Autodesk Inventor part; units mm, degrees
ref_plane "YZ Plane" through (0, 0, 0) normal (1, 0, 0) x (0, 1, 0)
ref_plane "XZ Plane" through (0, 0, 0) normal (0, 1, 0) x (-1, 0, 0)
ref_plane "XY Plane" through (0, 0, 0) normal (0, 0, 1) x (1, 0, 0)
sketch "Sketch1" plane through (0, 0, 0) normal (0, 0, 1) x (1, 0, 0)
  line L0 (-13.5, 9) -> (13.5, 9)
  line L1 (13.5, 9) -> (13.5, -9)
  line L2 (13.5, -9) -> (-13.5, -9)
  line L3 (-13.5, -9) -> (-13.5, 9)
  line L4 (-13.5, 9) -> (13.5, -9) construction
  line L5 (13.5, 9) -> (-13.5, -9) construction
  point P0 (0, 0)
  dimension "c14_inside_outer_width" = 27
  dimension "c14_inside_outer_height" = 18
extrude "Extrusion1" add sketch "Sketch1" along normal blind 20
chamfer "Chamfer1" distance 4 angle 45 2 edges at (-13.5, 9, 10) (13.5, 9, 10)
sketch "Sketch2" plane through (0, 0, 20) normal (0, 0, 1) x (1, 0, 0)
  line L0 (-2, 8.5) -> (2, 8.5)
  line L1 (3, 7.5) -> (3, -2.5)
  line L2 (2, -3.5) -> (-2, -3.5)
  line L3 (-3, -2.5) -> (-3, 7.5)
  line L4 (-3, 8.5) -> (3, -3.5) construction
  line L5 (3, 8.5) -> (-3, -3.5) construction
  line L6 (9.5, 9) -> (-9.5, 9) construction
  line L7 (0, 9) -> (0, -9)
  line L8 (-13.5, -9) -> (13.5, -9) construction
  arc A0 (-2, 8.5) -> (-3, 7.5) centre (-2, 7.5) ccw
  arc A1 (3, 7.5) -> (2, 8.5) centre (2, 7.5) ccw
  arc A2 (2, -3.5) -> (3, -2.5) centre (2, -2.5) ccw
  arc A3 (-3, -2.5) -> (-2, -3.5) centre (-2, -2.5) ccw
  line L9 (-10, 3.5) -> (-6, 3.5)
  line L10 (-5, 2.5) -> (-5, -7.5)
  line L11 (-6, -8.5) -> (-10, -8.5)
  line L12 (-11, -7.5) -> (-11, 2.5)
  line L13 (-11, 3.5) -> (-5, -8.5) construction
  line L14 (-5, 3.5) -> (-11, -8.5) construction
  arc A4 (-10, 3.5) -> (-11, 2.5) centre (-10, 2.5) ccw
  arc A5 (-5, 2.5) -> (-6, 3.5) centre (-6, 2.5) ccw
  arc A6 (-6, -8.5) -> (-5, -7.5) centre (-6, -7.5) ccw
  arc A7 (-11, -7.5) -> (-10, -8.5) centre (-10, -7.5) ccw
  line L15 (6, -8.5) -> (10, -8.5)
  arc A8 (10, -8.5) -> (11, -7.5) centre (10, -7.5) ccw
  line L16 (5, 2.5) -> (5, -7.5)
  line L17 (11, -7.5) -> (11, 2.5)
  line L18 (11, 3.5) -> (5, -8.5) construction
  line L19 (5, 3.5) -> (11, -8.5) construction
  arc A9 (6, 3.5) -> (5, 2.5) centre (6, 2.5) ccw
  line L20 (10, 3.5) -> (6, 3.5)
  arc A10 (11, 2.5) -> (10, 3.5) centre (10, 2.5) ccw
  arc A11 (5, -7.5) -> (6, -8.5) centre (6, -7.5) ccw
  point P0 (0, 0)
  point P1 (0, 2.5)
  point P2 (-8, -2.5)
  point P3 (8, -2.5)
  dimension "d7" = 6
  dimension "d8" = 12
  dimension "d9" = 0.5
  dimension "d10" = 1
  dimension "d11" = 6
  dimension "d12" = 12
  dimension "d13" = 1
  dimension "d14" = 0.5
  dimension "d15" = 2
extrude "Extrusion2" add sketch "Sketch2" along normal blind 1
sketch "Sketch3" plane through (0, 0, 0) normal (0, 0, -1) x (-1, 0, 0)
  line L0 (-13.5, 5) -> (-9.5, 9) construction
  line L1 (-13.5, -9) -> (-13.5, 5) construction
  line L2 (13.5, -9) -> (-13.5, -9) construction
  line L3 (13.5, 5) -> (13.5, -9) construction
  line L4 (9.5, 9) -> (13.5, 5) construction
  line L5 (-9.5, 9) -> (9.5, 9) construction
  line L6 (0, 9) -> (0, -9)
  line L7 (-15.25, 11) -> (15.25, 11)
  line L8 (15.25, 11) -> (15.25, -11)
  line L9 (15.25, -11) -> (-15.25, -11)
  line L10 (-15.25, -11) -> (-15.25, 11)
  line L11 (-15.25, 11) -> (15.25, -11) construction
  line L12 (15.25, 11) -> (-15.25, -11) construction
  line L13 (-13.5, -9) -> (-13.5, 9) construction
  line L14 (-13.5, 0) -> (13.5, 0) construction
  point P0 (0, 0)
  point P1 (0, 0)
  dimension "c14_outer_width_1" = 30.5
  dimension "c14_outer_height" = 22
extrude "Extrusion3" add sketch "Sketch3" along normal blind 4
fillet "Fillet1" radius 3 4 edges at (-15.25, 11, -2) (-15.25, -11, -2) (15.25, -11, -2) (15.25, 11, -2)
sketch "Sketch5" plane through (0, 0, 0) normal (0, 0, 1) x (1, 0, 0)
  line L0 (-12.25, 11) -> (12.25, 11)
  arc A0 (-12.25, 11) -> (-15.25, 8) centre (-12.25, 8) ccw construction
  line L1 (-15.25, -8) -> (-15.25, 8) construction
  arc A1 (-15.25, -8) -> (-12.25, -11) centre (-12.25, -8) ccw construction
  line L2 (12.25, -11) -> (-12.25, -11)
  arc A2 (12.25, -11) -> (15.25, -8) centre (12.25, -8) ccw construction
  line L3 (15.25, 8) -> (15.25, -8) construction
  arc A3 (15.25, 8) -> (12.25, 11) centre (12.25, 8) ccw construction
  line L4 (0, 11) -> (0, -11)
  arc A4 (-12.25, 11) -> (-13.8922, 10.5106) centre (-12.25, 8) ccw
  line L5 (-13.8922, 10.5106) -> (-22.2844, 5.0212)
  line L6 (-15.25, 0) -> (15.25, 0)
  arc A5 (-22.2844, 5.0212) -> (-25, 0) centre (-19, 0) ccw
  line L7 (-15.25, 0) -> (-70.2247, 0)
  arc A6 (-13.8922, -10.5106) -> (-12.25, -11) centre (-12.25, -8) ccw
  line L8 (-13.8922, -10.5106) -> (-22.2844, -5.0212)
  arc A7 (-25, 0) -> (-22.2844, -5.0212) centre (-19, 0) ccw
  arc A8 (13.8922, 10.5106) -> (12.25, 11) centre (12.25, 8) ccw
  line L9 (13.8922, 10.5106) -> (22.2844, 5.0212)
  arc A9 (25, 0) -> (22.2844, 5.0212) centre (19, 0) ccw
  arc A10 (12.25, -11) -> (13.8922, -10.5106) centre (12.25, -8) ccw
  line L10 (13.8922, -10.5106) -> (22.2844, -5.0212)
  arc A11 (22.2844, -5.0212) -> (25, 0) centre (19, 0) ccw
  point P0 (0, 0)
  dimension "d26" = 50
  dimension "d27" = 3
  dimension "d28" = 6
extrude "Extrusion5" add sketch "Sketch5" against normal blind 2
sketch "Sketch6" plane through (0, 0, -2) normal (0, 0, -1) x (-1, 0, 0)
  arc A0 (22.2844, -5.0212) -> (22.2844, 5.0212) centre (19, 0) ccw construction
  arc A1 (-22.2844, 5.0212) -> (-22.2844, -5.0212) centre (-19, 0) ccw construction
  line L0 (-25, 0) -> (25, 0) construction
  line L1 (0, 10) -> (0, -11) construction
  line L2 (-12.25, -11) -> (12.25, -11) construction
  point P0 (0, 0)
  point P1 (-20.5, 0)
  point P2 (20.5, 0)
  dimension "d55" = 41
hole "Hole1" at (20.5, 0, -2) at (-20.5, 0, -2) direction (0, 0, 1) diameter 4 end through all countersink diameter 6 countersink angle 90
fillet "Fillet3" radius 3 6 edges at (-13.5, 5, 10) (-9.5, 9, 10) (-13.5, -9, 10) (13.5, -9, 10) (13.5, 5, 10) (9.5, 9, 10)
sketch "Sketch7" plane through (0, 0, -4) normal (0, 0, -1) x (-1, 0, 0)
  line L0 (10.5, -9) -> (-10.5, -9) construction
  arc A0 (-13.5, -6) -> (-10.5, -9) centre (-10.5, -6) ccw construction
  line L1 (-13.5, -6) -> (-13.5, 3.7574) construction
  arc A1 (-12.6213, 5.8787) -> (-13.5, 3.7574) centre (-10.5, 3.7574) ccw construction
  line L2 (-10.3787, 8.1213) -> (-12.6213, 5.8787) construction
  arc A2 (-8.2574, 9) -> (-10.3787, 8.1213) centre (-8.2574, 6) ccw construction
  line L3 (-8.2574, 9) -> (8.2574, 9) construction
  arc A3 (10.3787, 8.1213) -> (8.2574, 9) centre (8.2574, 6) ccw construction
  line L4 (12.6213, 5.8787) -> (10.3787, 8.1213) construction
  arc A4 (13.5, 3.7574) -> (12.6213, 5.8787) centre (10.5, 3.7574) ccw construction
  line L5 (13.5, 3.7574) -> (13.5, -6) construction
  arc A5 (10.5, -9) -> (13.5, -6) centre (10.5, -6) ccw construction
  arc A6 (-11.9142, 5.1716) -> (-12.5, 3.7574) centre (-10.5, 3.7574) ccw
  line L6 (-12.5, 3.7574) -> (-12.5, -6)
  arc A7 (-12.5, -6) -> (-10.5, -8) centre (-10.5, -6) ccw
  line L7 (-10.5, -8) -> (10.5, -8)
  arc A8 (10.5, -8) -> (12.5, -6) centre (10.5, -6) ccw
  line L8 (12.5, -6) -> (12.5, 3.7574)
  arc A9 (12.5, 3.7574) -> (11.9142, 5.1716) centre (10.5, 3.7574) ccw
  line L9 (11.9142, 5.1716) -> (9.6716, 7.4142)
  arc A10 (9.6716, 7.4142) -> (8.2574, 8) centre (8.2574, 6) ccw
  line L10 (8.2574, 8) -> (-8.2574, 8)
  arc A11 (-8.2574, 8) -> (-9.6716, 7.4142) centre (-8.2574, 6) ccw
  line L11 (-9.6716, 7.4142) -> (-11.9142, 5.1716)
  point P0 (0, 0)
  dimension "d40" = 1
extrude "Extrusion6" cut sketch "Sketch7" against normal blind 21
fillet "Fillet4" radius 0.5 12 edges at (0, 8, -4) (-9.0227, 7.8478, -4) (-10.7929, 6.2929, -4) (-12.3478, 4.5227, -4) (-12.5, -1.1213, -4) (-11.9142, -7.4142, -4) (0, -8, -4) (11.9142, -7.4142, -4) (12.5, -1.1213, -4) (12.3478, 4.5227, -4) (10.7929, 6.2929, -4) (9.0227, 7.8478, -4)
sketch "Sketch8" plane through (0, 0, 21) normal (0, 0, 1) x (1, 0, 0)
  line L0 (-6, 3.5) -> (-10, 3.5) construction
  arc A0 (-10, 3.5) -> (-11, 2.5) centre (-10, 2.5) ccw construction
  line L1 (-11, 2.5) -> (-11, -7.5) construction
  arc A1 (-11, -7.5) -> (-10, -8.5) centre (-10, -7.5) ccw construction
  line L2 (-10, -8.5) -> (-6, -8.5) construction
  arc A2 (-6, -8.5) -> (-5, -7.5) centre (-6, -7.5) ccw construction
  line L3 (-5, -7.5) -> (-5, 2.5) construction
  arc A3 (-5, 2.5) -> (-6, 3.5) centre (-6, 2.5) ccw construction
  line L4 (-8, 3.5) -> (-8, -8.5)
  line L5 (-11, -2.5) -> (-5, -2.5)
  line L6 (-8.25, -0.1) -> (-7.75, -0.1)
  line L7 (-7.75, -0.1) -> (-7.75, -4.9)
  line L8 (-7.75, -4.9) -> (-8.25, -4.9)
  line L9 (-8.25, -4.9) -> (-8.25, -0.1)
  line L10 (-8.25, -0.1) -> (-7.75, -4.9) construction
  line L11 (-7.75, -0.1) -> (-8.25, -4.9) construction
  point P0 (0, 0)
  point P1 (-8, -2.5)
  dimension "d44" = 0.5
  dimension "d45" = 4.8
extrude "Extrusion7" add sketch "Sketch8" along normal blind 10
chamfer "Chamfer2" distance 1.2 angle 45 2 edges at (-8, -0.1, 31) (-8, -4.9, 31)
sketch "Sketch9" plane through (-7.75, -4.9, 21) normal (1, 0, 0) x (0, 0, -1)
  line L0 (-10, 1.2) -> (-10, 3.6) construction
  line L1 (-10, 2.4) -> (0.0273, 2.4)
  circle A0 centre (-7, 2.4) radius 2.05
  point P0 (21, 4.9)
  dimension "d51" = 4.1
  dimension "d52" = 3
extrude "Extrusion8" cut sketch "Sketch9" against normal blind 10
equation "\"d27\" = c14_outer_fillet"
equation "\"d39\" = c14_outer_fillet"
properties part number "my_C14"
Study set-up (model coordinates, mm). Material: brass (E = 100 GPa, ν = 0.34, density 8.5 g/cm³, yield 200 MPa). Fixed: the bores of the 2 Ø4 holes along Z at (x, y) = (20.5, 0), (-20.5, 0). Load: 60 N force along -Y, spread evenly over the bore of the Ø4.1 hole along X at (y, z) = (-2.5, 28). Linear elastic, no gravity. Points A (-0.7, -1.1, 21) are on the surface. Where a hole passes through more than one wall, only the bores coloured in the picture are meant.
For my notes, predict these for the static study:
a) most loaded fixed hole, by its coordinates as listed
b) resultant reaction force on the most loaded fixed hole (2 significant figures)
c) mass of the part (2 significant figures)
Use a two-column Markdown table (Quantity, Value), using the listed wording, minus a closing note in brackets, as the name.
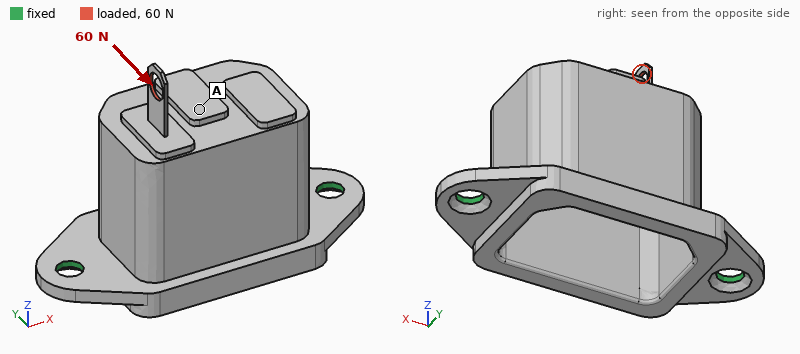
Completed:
| Quantity | Value |
|---|---|
| most loaded fixed hole, by its coordinates as listed | (-20.5, 0) |
| resultant reaction force on the most loaded fixed hole | 38 N |
| mass of the part | 38 g |
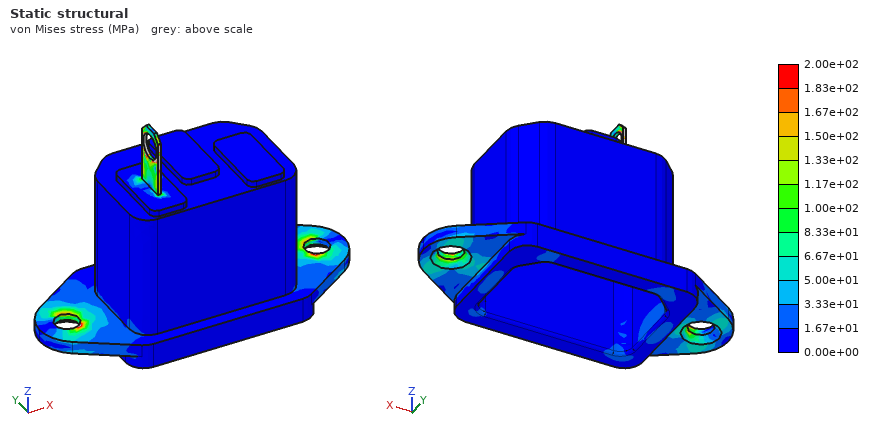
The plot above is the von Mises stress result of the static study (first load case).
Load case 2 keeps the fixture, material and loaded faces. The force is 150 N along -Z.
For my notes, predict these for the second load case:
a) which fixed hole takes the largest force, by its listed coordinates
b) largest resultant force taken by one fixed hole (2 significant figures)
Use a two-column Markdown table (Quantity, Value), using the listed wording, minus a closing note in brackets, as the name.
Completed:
| Quantity | Value |
|---|---|
| which fixed hole takes the largest force, by its listed coordinates | (-20.5, 0) |
| largest resultant force taken by one fixed hole | 110 N |
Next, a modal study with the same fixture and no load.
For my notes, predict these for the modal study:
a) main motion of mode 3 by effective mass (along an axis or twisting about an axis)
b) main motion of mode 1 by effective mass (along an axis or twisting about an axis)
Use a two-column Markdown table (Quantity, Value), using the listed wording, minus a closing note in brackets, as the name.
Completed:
| Quantity | Value |
|---|---|
| main motion of mode 3 by effective mass | along X |
| main motion of mode 1 by effective mass | along Y |
